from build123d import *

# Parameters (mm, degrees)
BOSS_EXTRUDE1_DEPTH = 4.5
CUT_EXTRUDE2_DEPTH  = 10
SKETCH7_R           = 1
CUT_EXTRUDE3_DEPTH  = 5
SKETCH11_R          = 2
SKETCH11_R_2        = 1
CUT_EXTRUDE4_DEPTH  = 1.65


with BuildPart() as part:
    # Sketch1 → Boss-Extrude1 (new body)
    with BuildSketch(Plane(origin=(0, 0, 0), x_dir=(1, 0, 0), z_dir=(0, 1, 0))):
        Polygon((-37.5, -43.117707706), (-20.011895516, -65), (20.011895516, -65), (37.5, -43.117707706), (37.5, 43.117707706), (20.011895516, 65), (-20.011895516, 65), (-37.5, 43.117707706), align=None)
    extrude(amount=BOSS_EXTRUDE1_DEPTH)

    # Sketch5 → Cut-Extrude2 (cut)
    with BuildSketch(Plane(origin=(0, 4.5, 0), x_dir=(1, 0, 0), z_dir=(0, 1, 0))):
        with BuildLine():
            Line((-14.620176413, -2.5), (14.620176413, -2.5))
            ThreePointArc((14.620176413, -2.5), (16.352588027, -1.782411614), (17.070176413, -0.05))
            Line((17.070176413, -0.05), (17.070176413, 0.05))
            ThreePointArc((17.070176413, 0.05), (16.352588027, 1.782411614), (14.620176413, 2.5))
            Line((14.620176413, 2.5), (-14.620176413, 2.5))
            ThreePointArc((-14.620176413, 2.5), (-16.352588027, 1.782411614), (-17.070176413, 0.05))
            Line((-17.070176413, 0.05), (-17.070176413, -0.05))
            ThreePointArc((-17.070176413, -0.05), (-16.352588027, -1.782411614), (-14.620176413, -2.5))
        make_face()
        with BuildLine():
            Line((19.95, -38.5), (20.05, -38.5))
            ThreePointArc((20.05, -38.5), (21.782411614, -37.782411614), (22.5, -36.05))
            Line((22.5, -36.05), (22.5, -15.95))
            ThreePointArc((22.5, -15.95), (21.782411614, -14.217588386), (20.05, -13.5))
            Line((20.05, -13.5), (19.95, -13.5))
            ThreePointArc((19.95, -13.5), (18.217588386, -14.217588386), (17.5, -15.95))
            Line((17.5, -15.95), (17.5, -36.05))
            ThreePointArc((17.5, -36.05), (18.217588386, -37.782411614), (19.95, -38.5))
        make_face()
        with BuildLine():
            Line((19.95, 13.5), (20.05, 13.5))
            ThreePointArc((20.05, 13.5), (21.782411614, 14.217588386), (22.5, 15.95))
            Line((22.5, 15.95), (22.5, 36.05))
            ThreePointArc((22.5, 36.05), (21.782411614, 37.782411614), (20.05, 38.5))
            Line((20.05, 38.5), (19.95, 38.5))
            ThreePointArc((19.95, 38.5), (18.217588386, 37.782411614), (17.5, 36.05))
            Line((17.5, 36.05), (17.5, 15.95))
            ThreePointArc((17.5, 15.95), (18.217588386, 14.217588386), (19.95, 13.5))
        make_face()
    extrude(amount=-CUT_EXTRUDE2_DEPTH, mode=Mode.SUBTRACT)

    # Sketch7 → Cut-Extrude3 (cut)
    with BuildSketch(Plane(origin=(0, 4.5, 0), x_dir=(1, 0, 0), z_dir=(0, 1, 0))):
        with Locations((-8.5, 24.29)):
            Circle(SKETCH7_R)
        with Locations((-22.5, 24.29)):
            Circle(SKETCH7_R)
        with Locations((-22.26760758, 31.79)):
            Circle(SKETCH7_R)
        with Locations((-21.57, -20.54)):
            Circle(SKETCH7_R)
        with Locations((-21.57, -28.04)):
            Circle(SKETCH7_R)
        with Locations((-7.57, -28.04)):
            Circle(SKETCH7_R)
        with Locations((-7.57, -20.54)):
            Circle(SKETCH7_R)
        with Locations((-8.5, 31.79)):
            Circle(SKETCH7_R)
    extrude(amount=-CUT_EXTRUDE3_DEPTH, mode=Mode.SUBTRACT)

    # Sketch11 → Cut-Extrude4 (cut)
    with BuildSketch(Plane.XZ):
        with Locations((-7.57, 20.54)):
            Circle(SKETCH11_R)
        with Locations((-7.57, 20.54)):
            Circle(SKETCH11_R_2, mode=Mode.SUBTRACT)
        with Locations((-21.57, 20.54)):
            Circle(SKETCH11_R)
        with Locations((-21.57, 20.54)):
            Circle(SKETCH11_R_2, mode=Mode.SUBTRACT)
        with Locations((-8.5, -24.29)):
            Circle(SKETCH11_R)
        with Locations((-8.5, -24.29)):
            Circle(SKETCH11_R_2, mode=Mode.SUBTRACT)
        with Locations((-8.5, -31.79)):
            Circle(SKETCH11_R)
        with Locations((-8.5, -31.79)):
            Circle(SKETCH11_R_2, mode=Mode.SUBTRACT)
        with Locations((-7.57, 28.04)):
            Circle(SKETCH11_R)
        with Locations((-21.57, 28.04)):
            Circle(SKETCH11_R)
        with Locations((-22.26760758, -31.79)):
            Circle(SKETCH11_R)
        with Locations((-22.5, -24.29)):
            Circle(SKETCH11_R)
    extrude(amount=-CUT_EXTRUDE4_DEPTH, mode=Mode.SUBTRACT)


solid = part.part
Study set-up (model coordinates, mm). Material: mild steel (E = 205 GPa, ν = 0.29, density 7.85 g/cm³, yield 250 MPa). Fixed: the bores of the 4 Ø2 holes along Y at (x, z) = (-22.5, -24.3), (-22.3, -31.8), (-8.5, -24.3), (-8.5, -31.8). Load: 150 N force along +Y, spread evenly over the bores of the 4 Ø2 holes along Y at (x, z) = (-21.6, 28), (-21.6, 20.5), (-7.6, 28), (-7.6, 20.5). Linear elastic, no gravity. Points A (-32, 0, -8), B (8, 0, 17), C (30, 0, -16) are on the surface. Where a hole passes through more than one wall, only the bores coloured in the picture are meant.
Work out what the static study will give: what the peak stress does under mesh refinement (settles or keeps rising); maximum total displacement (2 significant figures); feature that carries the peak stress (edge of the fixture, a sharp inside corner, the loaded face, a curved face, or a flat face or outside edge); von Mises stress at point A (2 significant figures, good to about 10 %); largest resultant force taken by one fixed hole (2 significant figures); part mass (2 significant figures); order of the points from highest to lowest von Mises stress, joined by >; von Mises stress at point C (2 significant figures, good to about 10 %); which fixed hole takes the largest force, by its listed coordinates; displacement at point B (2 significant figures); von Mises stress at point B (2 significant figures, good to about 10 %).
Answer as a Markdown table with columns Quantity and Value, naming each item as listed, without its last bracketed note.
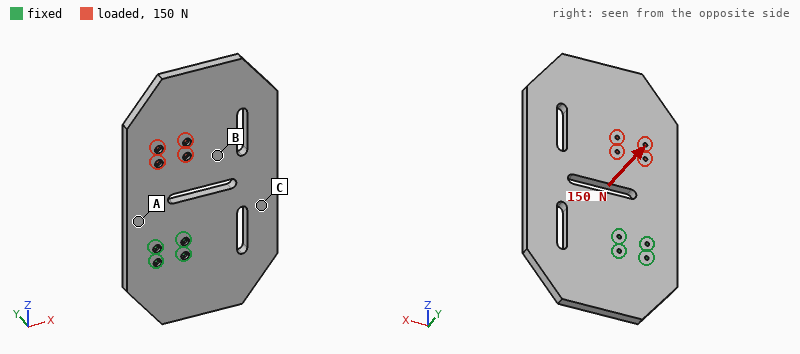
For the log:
| Quantity | Value |
|---|---|
| what the peak stress does under mesh refinement | keeps rising |
| maximum total displacement | 0.20 mm |
| feature that carries the peak stress | edge of the fixture |
| von Mises stress at point A | 32 MPa |
| largest resultant force taken by one fixed hole | 450 N |
| part mass | 300 g |
| order of the points from highest to lowest von Mises stress, joined by > | A > C > B |
| von Mises stress at point C | 17 MPa |
| which fixed hole takes the largest force, by its listed coordinates | (-8.5, -24.3) |
| displacement at point B | 0.073 mm |
| von Mises stress at point B | 6.6 MPa |
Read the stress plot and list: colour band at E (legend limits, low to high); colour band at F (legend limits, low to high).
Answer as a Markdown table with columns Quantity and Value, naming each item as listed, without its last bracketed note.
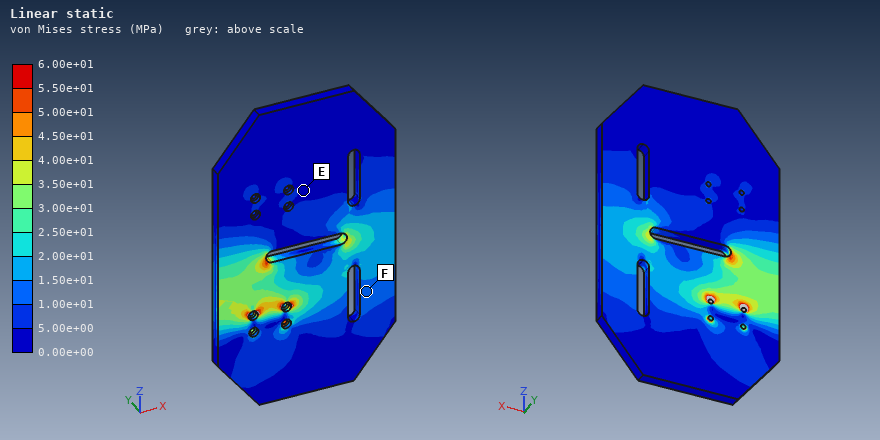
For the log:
| Quantity | Value |
|---|---|
| colour band at E | 0.00e+00 to 5.00e+00 MPa |
| colour band at F | 1.00e+01 to 1.50e+01 MPa |
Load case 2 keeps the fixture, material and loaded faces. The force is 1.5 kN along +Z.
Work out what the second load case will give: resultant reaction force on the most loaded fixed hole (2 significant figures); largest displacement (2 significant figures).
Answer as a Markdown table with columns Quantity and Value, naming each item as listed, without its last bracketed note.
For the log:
| Quantity | Value |
|---|---|
| resultant reaction force on the most loaded fixed hole | 490 N |
| largest displacement | 51 µm |
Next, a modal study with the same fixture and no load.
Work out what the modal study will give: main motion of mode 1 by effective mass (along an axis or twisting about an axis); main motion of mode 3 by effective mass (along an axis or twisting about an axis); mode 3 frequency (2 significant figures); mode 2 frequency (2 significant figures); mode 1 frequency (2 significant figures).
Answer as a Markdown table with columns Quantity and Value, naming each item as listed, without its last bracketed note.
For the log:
| Quantity | Value |
|---|---|
| main motion of mode 1 by effective mass | along Y |
| main motion of mode 3 by effective mass | along Y |
| mode 3 frequency | 1800 Hz |
| mode 2 frequency | 1000 Hz |
| mode 1 frequency | 380 Hz |
